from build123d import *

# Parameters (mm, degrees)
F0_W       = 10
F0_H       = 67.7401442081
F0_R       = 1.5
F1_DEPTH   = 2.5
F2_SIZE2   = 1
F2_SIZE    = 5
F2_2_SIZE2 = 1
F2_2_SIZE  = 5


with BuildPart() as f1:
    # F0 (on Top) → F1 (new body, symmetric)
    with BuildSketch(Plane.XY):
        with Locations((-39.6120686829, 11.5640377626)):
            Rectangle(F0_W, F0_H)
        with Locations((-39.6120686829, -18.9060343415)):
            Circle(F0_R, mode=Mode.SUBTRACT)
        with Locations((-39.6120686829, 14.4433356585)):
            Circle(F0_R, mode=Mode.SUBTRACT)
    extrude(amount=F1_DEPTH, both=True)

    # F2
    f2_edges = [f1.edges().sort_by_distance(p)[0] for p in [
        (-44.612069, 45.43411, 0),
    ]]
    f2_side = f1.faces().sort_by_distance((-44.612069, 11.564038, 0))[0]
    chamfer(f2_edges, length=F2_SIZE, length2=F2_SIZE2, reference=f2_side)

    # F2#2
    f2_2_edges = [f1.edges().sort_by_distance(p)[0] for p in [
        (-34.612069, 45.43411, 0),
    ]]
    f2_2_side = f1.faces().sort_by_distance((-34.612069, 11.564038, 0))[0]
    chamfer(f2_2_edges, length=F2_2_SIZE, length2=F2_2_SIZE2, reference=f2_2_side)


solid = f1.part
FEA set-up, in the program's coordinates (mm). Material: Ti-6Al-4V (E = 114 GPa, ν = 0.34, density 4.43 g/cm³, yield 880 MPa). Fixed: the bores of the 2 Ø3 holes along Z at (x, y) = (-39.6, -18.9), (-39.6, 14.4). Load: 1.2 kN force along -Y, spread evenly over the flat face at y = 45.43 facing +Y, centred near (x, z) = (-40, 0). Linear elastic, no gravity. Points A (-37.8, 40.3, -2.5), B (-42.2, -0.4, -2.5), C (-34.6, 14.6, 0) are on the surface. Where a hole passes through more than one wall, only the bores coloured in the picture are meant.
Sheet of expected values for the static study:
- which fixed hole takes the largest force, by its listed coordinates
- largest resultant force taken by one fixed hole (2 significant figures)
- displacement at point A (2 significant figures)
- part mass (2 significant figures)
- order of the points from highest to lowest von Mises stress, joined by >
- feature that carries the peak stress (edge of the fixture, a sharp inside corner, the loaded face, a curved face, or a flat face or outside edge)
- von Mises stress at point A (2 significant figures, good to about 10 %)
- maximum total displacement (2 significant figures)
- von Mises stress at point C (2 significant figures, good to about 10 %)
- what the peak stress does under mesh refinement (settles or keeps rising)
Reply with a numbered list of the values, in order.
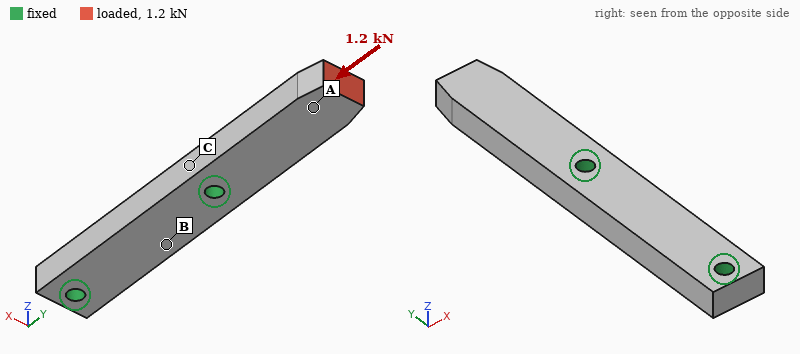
1. (-39.6, 14.4)
2. 1.2 kN
3. 5.7 µm
4. 15 g
5. A > C > B
6. edge of the fixture
7. 27 MPa
8. 7.0 µm
9. 12 MPa
10. keeps rising
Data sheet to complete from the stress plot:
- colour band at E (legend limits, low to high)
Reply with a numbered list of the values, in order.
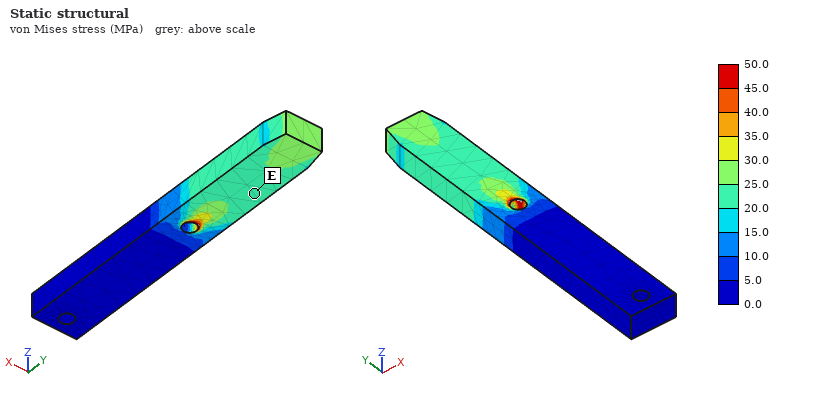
1. 20.0 to 25.0 MPa
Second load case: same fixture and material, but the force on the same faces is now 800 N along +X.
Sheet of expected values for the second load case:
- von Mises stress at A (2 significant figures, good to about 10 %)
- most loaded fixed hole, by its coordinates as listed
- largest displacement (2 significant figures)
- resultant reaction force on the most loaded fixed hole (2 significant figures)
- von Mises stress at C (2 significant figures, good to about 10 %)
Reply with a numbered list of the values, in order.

1. 42 MPa
2. (-39.6, 14.4)
3. 0.25 mm
4. 1.1 kN
5. 210 MPa
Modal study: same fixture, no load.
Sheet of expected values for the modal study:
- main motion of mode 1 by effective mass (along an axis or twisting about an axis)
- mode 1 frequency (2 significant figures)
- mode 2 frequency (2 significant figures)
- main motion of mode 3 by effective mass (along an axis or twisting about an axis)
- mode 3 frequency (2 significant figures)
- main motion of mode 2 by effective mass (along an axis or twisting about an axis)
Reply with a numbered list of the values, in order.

1. along Z
2. 4400 Hz
3. 6800 Hz
4. twisting about Y
5. 20 kHz
6. along X
